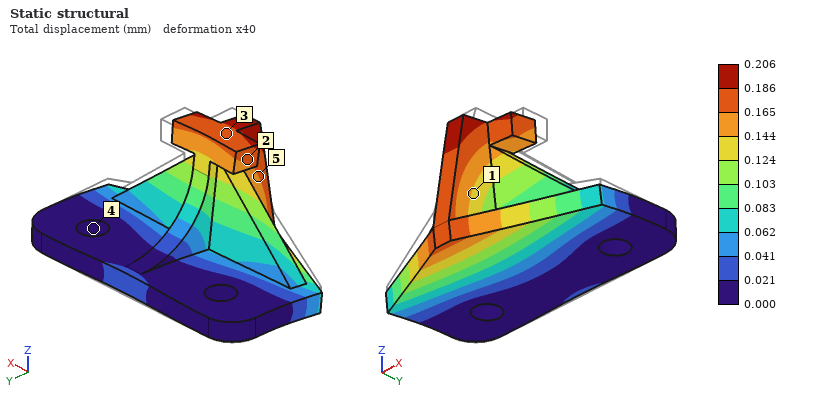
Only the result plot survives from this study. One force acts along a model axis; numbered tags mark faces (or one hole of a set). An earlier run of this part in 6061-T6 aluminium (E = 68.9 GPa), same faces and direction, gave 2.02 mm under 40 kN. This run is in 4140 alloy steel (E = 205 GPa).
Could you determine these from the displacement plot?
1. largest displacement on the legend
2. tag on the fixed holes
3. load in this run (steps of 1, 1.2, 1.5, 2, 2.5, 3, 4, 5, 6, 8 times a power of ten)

0.206 mm
4
12 kN
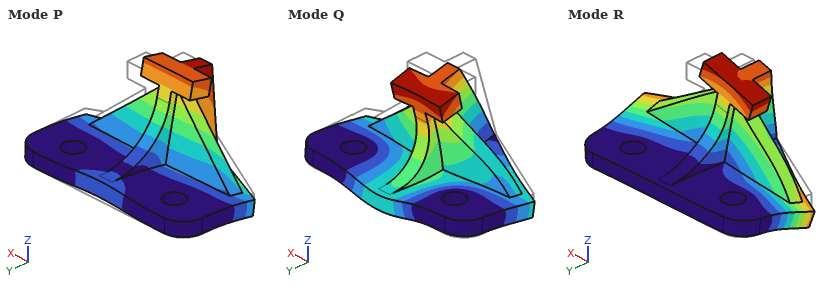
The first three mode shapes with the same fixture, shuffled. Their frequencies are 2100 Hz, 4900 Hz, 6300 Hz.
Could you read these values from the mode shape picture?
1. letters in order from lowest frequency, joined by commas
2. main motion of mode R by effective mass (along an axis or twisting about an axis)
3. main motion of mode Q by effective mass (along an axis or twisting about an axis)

P, R, Q
along X
along Z
